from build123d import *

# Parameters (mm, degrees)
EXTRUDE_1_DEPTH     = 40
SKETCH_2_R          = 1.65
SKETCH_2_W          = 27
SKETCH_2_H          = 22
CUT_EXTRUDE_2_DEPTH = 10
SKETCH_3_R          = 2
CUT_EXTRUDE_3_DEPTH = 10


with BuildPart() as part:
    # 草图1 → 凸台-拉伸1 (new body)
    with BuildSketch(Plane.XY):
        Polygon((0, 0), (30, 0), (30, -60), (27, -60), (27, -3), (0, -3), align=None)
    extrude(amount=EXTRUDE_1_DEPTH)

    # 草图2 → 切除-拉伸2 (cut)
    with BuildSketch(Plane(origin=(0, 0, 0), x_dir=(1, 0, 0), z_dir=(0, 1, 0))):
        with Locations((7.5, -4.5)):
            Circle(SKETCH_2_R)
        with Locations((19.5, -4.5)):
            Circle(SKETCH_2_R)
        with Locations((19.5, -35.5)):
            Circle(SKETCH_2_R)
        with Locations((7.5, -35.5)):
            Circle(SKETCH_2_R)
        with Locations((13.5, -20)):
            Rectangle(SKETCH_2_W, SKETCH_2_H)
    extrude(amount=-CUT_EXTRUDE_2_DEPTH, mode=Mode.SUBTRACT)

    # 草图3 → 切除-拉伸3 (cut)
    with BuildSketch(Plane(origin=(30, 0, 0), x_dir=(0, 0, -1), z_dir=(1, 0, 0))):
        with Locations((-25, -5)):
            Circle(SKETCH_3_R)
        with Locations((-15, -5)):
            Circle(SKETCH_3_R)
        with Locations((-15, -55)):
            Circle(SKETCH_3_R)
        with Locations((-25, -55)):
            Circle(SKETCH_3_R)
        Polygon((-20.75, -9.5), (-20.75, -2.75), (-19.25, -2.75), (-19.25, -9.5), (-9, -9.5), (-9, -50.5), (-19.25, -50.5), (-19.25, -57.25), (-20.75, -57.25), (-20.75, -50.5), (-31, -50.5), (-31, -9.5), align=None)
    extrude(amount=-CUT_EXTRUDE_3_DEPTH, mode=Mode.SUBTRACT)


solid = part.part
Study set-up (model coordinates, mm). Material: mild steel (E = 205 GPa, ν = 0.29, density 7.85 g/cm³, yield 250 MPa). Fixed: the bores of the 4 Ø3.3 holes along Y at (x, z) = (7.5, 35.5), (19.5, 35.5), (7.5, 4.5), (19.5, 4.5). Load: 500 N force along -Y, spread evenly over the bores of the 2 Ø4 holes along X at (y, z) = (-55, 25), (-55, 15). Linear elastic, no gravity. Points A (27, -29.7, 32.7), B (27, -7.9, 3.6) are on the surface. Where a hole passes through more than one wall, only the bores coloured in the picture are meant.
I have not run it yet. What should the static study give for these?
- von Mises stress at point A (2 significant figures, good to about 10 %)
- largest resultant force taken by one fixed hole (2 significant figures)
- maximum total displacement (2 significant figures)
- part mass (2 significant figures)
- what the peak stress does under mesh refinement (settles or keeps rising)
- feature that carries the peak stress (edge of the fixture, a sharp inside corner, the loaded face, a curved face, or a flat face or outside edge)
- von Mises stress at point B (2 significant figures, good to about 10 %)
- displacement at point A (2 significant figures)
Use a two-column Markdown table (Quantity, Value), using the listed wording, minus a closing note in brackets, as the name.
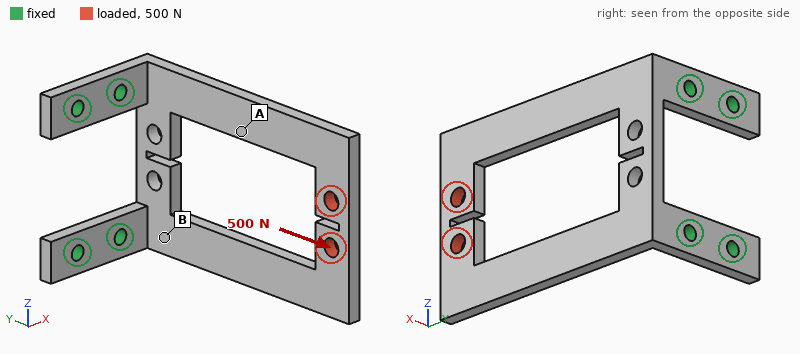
| Quantity | Value |
|---|---|
| von Mises stress at point A | 23 MPa |
| largest resultant force taken by one fixed hole | 260 N |
| maximum total displacement | 0.12 mm |
| part mass | 44 g |
| what the peak stress does under mesh refinement | keeps rising |
| feature that carries the peak stress | edge of the fixture |
| von Mises stress at point B | 11 MPa |
| displacement at point A | 0.058 mm |
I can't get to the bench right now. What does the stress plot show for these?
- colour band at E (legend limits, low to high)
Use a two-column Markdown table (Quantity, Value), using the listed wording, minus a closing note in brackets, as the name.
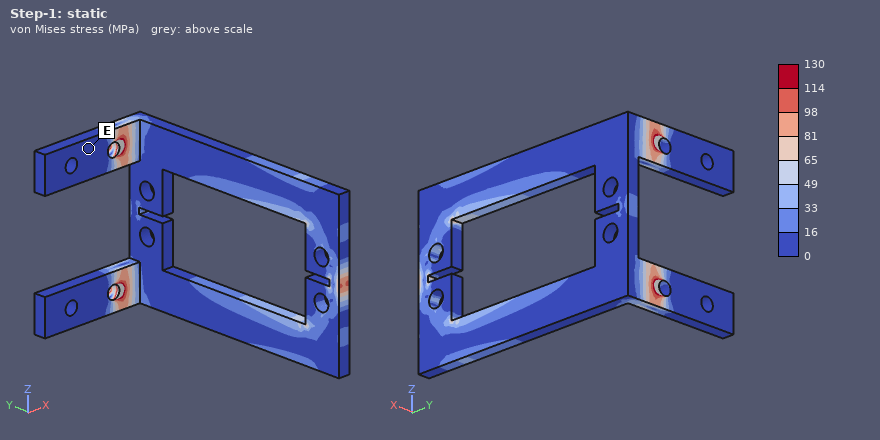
| Quantity | Value |
|---|---|
| colour band at E | 0 to 16 MPa |
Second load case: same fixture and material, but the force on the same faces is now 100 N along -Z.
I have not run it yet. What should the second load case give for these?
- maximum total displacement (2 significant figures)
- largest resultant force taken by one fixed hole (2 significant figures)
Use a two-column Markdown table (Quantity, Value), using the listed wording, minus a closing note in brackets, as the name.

| Quantity | Value |
|---|---|
| maximum total displacement | 47 µm |
| largest resultant force taken by one fixed hole | 170 N |
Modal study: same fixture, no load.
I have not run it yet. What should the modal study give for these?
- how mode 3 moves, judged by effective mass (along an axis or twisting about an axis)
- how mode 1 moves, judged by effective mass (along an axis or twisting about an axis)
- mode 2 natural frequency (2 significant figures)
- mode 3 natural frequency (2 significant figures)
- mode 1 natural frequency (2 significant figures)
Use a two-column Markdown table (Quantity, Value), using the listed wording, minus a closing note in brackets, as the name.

| Quantity | Value |
|---|---|
| how mode 3 moves, judged by effective mass | along Z |
| how mode 1 moves, judged by effective mass | along X |
| mode 2 natural frequency | 1500 Hz |
| mode 3 natural frequency | 2100 Hz |
| mode 1 natural frequency | 500 Hz |
